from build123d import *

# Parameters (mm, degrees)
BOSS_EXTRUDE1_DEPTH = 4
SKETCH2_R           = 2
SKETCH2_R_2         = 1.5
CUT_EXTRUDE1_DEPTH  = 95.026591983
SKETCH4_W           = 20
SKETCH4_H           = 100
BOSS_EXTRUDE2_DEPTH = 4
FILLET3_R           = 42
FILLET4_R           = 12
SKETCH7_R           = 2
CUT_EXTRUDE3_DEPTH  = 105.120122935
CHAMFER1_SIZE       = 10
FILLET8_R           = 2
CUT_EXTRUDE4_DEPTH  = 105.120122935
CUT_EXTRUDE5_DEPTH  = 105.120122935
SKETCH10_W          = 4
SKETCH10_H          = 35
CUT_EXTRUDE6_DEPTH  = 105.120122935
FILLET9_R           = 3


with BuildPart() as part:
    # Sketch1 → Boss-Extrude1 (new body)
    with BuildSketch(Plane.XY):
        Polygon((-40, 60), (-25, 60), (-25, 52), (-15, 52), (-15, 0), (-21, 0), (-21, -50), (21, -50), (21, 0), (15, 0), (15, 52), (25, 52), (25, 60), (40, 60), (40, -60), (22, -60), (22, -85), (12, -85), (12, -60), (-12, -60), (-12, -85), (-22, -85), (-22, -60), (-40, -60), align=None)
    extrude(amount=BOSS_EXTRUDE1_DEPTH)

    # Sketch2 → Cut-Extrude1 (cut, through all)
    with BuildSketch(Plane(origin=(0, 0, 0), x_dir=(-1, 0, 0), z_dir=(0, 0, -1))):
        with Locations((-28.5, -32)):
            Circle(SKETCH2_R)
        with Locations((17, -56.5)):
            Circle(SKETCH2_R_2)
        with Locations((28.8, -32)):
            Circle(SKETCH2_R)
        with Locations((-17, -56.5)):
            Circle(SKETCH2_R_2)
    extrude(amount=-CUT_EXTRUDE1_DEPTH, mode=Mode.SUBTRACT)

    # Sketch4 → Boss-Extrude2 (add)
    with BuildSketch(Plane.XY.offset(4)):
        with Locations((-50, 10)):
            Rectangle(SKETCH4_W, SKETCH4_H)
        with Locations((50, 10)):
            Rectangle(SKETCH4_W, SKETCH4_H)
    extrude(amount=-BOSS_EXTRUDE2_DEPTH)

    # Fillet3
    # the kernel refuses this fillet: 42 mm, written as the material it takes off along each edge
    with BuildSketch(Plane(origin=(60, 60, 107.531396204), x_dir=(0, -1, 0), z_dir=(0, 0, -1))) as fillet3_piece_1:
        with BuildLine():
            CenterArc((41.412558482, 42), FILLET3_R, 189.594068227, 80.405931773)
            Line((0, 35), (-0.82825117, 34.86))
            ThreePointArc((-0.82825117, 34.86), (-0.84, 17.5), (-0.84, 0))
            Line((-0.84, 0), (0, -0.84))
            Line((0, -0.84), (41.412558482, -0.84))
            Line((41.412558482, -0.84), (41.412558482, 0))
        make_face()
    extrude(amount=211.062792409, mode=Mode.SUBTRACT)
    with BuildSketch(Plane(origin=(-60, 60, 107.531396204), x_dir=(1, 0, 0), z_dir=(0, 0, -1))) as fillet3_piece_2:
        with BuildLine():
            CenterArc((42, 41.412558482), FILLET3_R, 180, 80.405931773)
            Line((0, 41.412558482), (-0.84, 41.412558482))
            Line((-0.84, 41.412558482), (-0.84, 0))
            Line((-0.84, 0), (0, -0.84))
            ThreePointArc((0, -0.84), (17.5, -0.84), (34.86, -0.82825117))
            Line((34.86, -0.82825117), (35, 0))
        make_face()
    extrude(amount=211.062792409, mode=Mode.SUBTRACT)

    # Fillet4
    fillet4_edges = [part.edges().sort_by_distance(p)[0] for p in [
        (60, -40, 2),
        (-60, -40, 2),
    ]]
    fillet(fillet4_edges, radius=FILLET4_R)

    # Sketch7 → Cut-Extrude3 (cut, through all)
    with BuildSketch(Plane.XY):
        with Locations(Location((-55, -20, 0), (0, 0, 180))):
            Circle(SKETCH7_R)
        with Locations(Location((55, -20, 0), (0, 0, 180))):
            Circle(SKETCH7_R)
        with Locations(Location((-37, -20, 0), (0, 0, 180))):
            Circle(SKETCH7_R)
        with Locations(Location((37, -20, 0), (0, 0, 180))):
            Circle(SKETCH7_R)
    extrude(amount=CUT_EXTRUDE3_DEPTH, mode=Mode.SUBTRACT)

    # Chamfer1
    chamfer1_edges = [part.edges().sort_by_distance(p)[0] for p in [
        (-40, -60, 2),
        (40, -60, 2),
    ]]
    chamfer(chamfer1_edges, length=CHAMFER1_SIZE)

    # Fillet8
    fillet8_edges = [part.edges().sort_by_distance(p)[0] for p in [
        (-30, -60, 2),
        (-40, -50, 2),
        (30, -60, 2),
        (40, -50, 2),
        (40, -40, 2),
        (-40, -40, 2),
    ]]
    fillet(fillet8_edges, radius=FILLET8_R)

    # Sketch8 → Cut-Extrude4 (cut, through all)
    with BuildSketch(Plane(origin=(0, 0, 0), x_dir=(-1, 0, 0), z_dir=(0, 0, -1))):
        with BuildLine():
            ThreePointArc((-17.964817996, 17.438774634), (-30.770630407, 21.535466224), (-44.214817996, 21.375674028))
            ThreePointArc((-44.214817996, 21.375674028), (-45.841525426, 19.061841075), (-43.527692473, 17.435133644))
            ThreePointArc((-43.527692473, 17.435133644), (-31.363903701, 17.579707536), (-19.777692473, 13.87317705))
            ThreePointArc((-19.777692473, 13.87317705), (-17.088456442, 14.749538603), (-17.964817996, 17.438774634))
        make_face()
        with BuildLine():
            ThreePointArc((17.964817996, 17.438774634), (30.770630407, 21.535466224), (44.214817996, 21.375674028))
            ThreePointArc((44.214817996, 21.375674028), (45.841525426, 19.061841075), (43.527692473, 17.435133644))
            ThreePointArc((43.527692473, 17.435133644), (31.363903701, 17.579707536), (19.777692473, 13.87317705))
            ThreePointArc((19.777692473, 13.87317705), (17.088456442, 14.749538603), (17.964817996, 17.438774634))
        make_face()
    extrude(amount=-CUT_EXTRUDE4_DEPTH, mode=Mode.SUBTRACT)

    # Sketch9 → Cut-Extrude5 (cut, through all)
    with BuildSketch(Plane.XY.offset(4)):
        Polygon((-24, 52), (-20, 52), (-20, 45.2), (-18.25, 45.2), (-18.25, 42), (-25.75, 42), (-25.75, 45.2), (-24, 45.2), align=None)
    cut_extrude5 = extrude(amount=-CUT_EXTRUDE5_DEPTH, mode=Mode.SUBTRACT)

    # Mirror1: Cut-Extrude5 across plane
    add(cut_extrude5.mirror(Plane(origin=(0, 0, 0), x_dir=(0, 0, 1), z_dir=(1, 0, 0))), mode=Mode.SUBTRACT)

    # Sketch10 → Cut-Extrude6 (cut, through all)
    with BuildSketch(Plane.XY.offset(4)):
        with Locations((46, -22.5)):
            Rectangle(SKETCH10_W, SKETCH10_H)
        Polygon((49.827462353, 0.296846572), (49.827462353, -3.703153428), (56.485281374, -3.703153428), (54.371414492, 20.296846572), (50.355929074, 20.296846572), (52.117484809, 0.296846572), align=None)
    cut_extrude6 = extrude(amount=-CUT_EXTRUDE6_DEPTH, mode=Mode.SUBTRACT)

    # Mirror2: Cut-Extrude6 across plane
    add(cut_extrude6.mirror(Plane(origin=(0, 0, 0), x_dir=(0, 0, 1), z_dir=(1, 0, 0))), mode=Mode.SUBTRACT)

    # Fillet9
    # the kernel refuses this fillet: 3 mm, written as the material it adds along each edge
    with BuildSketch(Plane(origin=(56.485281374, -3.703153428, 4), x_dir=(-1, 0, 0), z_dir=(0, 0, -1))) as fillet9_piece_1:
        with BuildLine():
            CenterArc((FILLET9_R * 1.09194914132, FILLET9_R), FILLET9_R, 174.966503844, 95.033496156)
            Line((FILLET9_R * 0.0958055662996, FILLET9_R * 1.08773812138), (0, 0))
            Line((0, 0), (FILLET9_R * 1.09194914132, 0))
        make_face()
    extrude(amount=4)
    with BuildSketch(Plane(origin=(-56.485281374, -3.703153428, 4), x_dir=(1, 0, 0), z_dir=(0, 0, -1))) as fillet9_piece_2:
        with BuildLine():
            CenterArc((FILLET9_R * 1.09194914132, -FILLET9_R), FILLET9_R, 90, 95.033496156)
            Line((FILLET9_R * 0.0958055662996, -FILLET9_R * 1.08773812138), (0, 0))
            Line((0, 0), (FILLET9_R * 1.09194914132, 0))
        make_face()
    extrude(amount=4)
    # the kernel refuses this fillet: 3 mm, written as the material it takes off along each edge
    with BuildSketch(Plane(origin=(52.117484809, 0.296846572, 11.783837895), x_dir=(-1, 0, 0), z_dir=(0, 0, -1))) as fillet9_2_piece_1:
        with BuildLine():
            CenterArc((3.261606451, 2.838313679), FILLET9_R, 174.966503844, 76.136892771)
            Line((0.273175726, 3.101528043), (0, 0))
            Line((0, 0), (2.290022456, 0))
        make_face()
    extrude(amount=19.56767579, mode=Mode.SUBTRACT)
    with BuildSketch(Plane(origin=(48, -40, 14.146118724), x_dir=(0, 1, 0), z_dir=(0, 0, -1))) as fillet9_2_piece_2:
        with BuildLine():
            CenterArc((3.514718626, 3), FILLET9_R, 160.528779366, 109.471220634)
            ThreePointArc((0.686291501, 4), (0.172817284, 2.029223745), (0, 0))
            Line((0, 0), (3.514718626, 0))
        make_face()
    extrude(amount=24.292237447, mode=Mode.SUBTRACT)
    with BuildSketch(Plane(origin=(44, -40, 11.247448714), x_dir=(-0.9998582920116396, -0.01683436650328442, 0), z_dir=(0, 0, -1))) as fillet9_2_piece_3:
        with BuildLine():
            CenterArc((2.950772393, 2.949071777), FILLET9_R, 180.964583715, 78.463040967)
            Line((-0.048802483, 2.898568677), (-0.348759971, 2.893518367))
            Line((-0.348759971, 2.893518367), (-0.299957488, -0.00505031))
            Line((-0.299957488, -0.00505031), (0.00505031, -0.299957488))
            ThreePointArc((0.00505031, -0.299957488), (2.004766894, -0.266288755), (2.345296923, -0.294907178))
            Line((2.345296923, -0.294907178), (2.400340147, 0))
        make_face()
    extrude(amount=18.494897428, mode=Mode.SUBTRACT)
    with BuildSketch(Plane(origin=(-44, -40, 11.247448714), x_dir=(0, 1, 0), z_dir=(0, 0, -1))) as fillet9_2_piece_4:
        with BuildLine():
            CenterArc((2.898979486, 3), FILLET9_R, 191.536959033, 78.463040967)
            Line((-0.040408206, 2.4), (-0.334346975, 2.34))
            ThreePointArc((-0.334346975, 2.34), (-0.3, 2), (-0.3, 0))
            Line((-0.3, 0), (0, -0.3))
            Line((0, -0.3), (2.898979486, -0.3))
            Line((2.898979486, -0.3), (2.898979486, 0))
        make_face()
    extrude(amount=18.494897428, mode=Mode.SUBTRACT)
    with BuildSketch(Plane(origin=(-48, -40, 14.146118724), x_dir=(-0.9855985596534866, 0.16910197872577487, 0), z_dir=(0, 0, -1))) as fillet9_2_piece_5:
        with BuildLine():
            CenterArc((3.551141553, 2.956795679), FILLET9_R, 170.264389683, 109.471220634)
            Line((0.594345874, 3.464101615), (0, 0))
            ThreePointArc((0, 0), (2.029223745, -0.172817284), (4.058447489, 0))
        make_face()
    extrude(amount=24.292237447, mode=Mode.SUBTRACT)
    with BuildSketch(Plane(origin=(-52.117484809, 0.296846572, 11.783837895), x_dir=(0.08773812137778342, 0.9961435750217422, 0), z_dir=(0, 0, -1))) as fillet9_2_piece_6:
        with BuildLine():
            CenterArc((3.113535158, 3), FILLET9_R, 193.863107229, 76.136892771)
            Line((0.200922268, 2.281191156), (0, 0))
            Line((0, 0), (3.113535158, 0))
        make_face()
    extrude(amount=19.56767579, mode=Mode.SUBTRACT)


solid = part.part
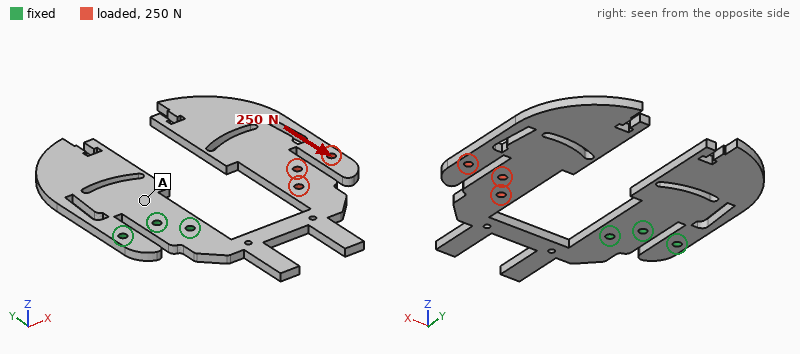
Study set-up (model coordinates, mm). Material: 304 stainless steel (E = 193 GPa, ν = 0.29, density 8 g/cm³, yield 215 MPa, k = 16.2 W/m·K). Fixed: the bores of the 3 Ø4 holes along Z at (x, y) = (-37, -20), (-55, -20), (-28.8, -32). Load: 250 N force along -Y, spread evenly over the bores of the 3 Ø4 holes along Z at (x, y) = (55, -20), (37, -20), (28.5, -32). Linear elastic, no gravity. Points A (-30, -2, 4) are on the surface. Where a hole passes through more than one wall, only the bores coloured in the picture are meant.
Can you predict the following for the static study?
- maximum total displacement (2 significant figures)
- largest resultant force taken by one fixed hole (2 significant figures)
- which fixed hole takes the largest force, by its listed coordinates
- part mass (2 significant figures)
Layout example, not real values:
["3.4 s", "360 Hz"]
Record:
["1.0 mm", "1.1 kN", "(-28.8, -32)", "260 g"]
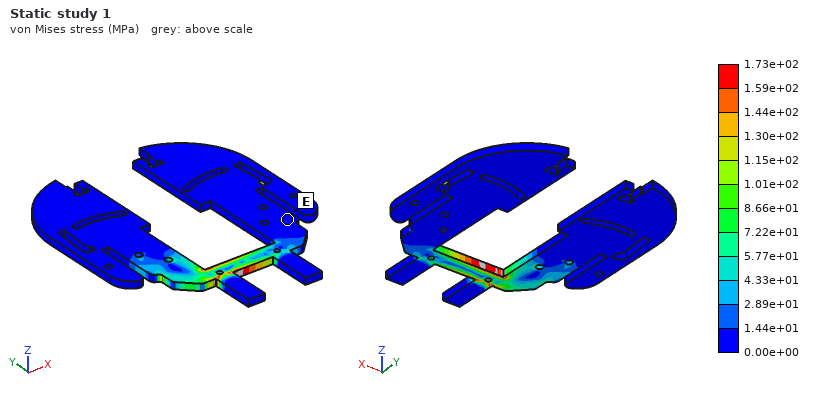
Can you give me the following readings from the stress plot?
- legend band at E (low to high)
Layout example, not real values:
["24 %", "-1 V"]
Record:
["0.00e+00 to 1.44e+01 MPa"]
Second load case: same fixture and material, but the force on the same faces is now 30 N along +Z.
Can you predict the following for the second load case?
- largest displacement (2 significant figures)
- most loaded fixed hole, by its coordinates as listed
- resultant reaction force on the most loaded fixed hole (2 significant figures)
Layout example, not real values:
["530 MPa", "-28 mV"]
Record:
["0.94 mm", "(-28.8, -32)", "38 N"]
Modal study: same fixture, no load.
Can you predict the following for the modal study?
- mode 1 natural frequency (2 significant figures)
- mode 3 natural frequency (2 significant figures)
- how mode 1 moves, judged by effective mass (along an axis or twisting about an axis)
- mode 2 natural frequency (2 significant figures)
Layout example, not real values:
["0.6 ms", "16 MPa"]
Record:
["79 Hz", "250 Hz", "along Z", "210 Hz"]
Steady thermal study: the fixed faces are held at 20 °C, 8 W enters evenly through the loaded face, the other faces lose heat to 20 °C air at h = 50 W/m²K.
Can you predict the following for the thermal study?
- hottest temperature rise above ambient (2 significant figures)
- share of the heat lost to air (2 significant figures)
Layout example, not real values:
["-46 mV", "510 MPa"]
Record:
["49 K", "100 %"]
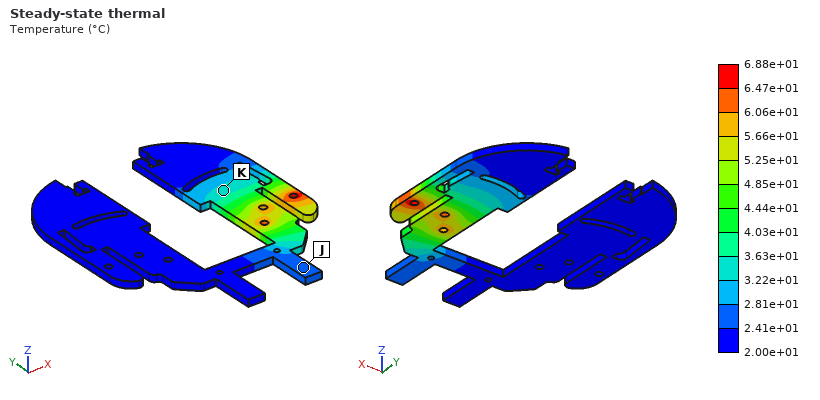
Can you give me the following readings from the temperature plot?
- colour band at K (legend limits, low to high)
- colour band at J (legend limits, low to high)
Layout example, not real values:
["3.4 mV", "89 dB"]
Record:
["3.22e+01 to 3.63e+01 °C", "2.41e+01 to 2.81e+01 °C"]
